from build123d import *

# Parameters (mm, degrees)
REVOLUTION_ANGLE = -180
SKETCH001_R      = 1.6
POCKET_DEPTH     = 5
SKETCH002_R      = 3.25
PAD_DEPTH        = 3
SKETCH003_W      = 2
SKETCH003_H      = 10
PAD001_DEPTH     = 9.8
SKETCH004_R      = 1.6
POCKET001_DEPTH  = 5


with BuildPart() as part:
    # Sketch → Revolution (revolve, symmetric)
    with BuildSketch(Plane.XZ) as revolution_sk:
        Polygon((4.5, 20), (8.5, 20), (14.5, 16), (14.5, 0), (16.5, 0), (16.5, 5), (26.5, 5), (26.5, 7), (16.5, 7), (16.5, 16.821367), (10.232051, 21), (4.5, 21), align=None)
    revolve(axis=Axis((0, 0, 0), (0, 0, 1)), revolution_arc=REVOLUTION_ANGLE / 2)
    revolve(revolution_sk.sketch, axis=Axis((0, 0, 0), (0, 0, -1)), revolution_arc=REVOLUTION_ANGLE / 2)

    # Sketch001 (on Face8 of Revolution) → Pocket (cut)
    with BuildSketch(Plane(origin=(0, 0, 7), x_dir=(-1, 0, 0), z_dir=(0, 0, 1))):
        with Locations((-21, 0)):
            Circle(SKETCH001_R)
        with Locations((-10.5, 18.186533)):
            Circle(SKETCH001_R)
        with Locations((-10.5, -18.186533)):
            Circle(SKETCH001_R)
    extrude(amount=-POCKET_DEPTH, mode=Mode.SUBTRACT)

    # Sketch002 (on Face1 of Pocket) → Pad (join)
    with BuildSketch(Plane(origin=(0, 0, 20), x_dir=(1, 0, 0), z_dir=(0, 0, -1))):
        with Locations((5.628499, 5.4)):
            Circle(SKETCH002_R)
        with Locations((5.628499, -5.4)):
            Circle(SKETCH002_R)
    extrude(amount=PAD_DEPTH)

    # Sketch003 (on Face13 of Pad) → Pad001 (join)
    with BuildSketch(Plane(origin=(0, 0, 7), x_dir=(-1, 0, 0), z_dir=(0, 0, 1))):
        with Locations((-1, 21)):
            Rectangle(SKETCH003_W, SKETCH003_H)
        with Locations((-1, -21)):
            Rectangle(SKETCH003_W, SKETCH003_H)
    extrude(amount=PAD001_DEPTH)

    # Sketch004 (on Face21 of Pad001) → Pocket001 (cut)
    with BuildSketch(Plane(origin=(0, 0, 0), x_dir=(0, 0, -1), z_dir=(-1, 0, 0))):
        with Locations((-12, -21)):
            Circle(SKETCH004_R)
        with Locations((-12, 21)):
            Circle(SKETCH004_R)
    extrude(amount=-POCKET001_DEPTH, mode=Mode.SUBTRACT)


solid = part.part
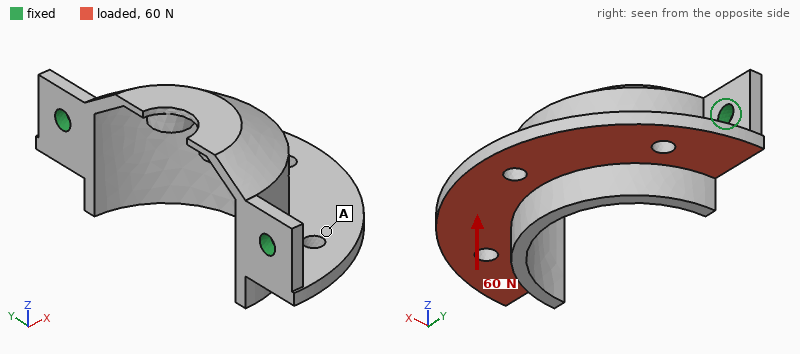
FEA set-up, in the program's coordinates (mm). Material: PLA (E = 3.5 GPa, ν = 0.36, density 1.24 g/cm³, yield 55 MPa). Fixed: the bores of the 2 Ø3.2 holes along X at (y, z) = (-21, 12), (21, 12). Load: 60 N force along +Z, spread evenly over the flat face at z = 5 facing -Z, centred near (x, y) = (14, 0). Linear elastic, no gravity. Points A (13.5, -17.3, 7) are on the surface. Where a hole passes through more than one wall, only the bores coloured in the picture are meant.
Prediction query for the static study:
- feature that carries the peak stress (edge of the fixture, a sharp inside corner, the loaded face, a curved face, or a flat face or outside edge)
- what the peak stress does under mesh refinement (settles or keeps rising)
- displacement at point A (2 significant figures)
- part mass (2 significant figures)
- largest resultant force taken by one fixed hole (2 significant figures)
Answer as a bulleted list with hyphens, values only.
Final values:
- edge of the fixture
- keeps rising
- 0.35 mm
- 5.0 g
- 30 N
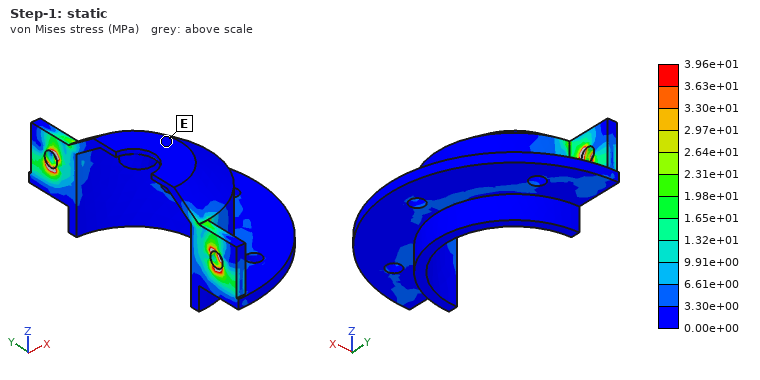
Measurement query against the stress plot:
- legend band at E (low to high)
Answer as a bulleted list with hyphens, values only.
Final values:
- 0.00e+00 to 3.30e+00 MPa
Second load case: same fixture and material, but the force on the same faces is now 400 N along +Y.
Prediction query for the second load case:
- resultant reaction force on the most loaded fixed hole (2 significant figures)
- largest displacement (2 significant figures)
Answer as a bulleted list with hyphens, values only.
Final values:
- 240 N
- 0.30 mm
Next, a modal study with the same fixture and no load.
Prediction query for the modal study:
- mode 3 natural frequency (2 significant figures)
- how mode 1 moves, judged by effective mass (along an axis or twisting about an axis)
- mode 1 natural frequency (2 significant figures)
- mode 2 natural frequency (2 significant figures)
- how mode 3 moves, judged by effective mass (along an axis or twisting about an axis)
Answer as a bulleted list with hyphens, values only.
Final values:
- 4300 Hz
- along Z
- 1000 Hz
- 3200 Hz
- along X
